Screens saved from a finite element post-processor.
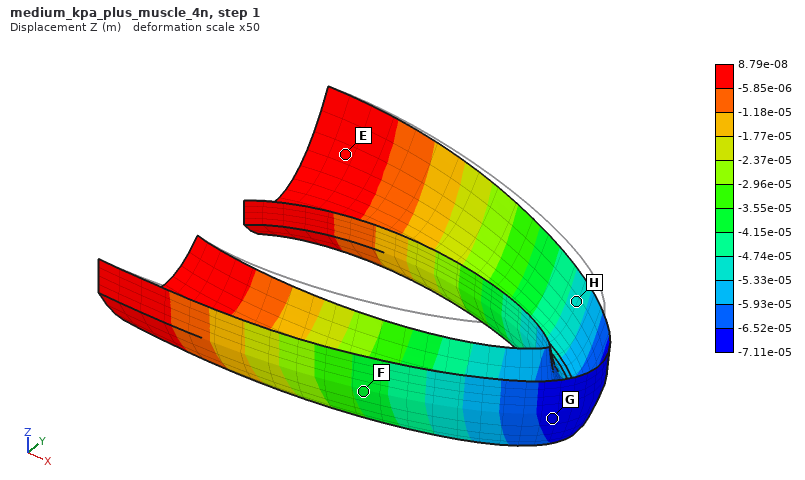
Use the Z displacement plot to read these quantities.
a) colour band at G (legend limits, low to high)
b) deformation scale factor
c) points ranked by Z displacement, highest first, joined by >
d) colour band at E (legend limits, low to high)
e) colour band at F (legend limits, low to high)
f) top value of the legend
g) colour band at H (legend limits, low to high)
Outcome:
-7.11e-05 to -6.52e-05 m
50
E > F > H > G
-5.85e-06 to 8.79e-08 m
-4.15e-05 to -3.55e-05 m
8.79e-08 m
-5.33e-05 to -4.74e-05 m
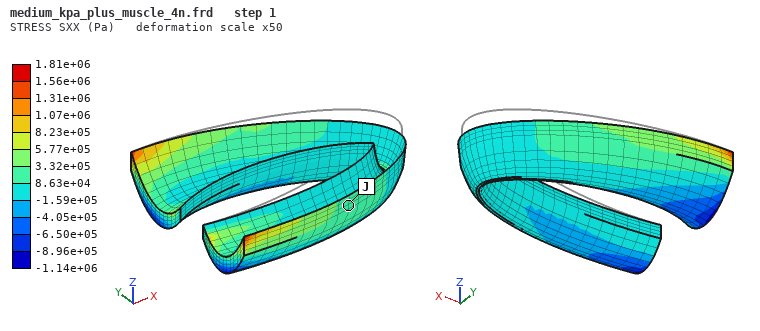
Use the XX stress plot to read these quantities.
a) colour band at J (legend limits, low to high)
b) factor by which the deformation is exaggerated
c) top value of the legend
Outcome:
8.63e+04 to 3.32e+05 Pa
50
1.81e+06 Pa
